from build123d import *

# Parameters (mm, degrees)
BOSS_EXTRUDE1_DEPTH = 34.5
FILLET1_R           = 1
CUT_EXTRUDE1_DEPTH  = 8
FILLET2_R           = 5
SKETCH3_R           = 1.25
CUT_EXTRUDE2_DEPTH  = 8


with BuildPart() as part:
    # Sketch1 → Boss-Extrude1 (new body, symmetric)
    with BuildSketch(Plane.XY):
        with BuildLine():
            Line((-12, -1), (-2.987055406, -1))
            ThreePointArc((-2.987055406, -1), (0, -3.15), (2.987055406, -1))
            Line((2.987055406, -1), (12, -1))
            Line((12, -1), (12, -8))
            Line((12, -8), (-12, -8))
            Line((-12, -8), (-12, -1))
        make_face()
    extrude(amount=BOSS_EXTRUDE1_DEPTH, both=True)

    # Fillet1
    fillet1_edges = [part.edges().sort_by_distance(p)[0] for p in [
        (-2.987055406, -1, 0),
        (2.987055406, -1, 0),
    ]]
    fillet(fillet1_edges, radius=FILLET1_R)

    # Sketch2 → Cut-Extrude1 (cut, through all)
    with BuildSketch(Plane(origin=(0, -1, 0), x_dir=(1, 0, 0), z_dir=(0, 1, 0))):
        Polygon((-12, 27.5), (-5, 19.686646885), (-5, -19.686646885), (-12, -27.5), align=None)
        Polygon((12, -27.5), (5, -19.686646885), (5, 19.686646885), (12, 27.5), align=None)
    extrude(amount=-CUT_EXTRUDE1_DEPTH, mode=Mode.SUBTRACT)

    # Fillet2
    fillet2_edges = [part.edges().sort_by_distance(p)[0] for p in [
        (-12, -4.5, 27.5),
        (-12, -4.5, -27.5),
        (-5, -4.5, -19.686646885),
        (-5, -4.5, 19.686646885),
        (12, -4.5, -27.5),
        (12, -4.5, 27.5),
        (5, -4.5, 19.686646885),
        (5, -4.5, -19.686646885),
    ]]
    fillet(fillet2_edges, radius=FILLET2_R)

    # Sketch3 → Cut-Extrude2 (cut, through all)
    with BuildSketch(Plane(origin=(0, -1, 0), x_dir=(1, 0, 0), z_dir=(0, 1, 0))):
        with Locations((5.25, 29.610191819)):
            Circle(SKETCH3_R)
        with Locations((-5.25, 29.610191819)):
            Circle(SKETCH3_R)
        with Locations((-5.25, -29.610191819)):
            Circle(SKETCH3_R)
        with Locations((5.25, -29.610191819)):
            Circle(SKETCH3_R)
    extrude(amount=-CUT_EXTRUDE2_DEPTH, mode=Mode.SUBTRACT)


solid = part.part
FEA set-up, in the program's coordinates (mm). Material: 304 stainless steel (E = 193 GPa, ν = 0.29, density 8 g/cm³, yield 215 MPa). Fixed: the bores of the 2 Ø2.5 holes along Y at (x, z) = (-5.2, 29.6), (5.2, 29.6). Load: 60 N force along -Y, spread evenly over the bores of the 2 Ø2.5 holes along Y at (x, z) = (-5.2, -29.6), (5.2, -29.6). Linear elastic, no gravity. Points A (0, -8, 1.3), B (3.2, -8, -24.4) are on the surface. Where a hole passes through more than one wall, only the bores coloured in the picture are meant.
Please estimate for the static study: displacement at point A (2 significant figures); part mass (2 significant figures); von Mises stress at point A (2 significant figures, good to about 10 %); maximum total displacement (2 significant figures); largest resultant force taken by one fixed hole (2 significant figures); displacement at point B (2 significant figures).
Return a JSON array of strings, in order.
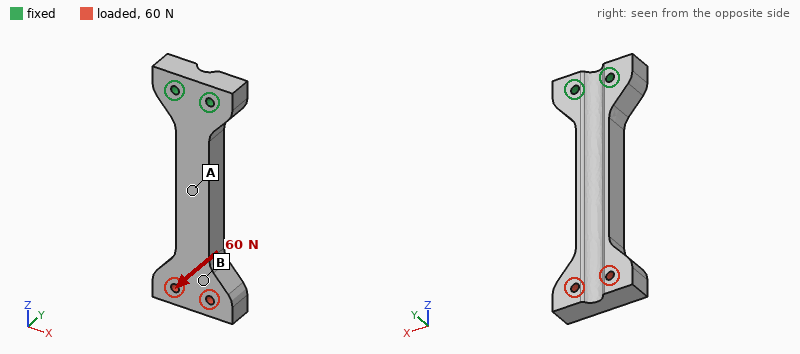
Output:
["23 µm", "49 g", "28 MPa", "98 µm", "31 N", "75 µm"]
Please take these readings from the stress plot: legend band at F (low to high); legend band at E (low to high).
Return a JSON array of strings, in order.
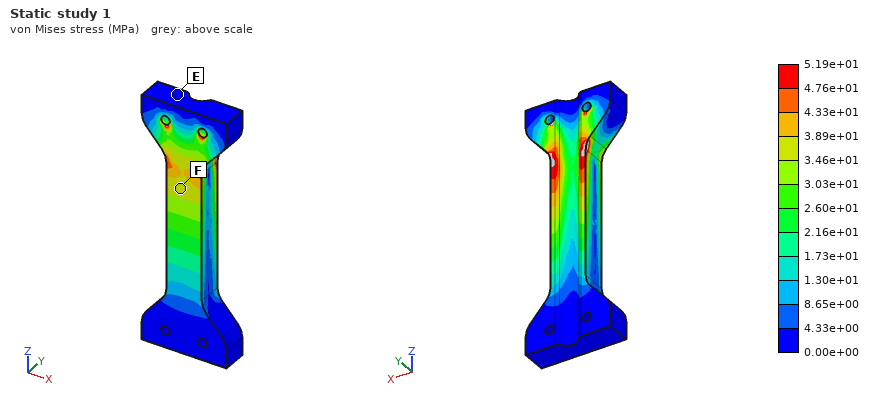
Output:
["3.46e+01 to 3.89e+01 MPa", "0.00e+00 to 4.33e+00 MPa"]
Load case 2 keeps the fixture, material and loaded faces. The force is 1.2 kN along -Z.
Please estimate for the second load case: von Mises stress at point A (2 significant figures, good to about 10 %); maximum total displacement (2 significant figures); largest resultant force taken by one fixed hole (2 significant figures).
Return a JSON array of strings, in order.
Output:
["12 MPa", "21 µm", "620 N"]
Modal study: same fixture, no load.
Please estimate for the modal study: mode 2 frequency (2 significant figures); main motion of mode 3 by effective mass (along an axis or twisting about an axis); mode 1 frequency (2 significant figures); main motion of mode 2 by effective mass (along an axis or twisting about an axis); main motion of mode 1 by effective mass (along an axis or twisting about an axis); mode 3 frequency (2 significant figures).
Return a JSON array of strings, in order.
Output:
["1800 Hz", "twisting about Z", "1000 Hz", "along X", "along Y", "4400 Hz"]
